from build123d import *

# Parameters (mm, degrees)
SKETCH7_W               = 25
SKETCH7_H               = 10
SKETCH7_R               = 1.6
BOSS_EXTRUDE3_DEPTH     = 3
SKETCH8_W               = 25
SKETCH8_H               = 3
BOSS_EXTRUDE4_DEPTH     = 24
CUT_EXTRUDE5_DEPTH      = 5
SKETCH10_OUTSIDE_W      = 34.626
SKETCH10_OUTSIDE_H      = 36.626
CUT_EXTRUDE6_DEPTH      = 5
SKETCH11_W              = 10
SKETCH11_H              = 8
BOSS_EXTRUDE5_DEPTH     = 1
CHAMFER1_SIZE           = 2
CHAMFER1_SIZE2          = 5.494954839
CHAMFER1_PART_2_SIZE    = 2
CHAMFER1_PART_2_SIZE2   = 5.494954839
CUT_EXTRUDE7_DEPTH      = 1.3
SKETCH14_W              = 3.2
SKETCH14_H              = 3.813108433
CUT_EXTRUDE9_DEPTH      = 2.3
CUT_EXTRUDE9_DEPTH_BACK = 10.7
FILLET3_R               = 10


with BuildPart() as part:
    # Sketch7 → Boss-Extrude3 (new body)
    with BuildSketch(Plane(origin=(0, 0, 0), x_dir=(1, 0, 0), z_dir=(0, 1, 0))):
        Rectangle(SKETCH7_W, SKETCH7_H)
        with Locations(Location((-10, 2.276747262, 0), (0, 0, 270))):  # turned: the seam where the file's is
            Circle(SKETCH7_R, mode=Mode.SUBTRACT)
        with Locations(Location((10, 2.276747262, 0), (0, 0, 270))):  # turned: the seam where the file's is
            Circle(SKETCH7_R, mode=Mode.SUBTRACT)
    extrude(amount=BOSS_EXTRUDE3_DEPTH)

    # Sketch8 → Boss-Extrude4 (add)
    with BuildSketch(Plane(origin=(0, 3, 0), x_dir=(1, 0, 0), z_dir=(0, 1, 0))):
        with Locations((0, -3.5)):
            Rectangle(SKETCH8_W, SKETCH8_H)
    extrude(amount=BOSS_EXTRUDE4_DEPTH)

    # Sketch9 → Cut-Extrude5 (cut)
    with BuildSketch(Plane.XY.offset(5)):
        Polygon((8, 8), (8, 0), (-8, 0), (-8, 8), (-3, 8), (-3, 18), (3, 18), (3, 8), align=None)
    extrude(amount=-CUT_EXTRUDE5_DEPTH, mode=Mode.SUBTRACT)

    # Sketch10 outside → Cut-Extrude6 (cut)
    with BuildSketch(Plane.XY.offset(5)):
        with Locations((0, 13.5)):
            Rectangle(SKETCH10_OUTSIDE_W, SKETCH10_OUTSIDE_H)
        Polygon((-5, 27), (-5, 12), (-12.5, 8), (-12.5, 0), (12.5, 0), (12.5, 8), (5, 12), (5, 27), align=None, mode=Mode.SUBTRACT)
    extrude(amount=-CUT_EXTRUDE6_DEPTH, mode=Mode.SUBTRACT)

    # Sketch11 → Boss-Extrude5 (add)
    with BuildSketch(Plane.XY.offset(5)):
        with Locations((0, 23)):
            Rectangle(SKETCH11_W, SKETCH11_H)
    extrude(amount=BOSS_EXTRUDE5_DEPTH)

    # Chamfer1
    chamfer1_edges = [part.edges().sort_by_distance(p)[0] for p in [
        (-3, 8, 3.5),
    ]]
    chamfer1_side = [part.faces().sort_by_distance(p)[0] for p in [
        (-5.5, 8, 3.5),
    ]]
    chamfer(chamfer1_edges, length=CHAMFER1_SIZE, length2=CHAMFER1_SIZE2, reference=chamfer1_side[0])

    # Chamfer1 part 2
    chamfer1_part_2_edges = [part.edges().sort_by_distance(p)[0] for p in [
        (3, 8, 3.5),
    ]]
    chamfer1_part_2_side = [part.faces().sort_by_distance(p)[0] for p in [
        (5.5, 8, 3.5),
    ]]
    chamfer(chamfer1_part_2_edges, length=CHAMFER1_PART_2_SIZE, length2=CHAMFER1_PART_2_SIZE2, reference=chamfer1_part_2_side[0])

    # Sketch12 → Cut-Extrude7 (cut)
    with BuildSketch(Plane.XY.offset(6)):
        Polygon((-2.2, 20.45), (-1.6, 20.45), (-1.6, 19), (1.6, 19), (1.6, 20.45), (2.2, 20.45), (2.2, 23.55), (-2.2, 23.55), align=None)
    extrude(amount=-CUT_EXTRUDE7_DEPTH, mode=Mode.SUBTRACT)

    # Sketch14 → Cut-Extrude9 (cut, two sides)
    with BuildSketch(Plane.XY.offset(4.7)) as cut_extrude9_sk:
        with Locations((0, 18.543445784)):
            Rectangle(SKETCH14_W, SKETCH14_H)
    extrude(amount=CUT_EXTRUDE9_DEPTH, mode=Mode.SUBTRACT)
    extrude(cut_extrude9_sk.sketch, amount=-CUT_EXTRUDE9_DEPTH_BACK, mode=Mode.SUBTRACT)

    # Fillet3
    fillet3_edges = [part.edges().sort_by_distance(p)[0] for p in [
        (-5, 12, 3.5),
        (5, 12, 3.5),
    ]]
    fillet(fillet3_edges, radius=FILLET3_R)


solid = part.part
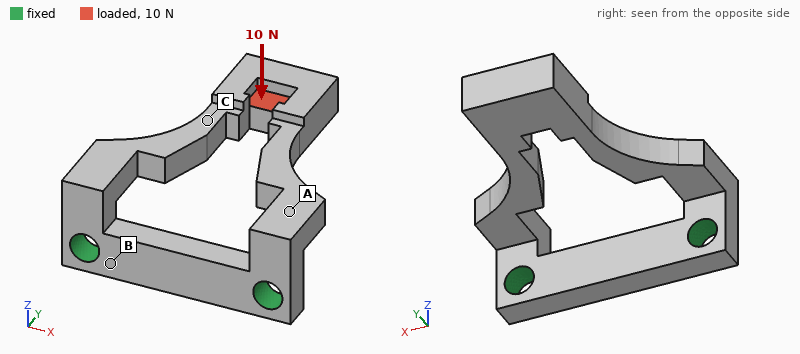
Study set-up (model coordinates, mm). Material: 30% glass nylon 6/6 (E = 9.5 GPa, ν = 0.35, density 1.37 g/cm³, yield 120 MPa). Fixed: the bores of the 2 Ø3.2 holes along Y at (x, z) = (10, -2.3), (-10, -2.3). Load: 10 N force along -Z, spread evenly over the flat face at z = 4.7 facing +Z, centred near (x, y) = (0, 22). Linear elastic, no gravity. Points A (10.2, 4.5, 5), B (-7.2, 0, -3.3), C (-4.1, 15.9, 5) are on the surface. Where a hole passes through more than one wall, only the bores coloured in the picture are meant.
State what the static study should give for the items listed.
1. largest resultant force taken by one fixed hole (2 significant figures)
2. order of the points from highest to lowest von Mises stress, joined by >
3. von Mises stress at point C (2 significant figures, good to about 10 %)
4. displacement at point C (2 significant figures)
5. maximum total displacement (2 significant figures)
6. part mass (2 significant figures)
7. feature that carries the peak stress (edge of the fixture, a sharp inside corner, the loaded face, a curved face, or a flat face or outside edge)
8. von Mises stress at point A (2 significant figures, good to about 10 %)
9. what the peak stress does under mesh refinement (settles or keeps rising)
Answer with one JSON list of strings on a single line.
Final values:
["5.0 N", "A > C > B", "9.3 MPa", "0.19 mm", "0.44 mm", "1.5 g", "a sharp inside corner", "14 MPa", "keeps rising"]
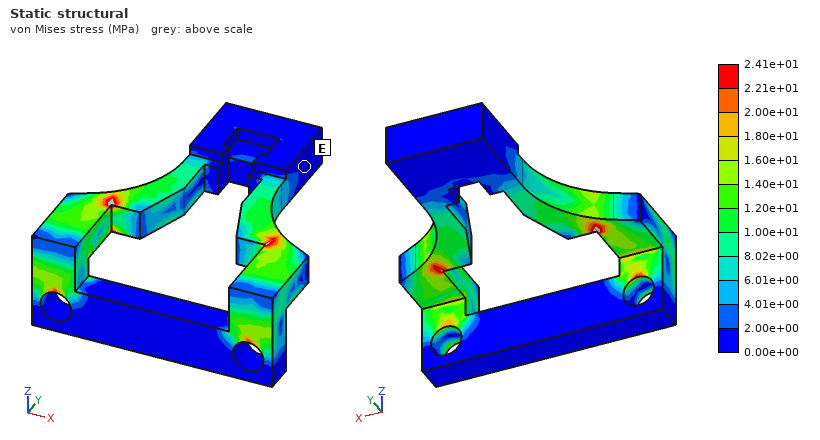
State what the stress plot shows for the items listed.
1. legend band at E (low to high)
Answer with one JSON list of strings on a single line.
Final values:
["0.00e+00 to 2.00e+00 MPa"]
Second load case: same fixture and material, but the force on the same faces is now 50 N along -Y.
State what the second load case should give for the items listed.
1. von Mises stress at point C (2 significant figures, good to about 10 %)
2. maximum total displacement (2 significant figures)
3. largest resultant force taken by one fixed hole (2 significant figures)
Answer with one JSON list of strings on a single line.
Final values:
["13 MPa", "0.27 mm", "27 N"]
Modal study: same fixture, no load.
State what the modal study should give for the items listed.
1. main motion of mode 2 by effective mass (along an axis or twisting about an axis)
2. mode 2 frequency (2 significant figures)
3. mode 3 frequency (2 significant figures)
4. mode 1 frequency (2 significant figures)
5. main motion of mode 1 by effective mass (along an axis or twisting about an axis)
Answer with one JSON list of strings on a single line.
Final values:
["along X", "4700 Hz", "5600 Hz", "1200 Hz", "along Z"]
